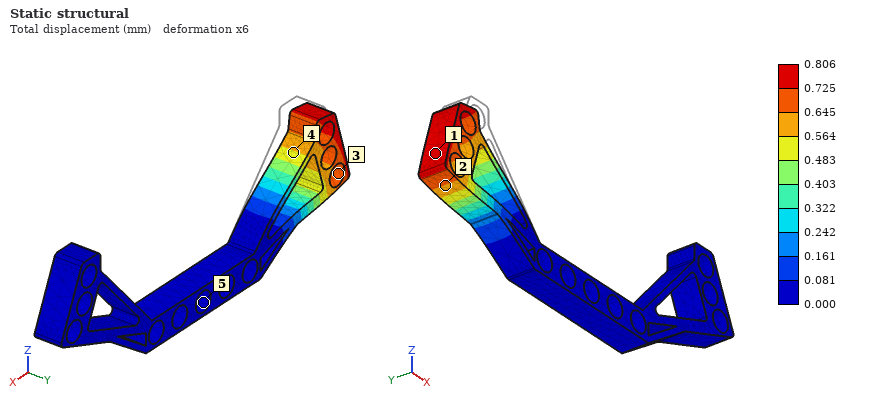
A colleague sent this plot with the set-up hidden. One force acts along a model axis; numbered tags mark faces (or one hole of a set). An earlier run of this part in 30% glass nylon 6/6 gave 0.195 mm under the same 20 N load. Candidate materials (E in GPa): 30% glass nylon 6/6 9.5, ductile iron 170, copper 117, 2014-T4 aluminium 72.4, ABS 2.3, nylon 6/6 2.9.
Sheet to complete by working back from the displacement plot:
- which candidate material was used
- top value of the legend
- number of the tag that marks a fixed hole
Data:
ABS
0.806 mm
5
